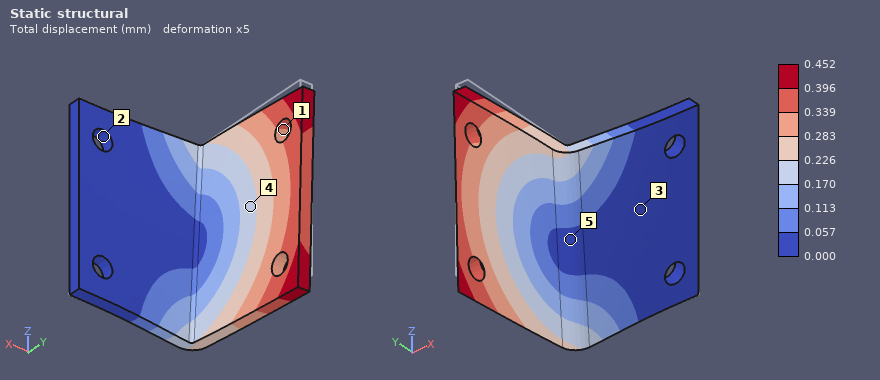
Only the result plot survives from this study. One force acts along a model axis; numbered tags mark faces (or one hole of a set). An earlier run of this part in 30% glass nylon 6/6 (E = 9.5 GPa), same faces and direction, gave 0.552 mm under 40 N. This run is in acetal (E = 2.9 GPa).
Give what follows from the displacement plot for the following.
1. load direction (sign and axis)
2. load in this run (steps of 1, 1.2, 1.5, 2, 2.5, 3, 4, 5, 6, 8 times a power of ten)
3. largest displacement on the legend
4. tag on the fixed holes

-Z
10 N
0.452 mm
2
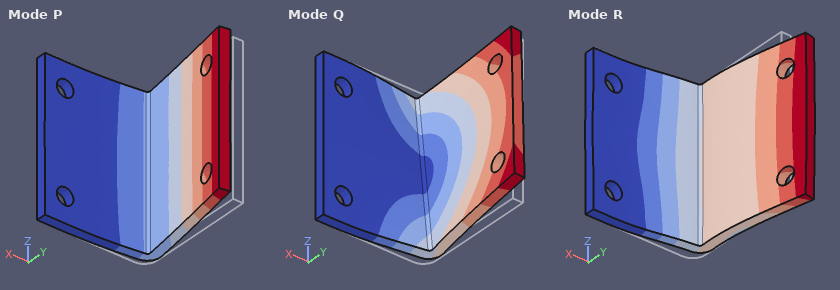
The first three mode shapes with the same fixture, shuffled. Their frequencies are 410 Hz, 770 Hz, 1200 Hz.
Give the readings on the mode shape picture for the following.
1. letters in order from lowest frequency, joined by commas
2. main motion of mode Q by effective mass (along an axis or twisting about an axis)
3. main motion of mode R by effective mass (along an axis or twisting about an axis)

P, Q, R
along Z
along Y
